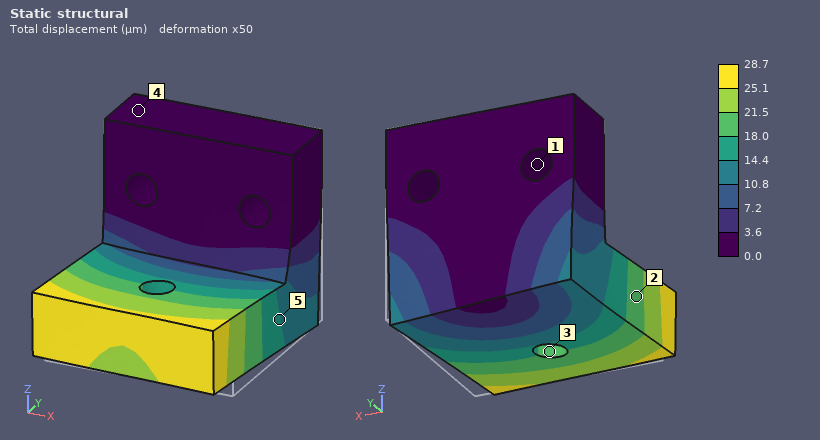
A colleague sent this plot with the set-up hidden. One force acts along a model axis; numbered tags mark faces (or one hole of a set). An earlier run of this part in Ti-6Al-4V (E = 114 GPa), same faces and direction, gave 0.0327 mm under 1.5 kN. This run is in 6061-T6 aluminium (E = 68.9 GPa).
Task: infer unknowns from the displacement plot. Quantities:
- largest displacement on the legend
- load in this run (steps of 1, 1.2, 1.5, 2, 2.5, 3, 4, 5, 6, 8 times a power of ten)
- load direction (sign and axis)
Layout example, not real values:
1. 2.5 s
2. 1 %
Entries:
1. 28.7 µm
2. 800 N
3. -X
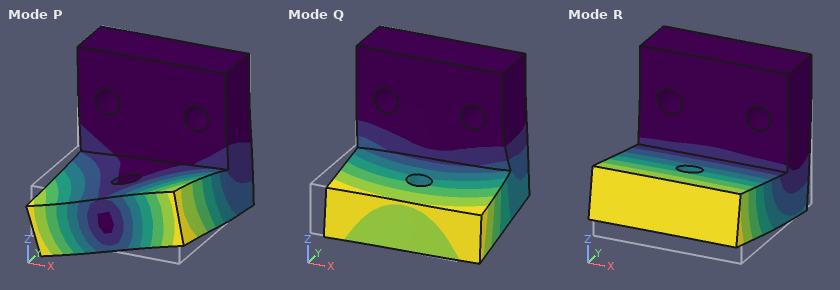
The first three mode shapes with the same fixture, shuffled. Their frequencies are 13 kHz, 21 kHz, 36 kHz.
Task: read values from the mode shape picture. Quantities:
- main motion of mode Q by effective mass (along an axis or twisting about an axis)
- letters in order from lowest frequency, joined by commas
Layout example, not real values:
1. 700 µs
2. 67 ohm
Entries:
1. along X
2. R, Q, P
